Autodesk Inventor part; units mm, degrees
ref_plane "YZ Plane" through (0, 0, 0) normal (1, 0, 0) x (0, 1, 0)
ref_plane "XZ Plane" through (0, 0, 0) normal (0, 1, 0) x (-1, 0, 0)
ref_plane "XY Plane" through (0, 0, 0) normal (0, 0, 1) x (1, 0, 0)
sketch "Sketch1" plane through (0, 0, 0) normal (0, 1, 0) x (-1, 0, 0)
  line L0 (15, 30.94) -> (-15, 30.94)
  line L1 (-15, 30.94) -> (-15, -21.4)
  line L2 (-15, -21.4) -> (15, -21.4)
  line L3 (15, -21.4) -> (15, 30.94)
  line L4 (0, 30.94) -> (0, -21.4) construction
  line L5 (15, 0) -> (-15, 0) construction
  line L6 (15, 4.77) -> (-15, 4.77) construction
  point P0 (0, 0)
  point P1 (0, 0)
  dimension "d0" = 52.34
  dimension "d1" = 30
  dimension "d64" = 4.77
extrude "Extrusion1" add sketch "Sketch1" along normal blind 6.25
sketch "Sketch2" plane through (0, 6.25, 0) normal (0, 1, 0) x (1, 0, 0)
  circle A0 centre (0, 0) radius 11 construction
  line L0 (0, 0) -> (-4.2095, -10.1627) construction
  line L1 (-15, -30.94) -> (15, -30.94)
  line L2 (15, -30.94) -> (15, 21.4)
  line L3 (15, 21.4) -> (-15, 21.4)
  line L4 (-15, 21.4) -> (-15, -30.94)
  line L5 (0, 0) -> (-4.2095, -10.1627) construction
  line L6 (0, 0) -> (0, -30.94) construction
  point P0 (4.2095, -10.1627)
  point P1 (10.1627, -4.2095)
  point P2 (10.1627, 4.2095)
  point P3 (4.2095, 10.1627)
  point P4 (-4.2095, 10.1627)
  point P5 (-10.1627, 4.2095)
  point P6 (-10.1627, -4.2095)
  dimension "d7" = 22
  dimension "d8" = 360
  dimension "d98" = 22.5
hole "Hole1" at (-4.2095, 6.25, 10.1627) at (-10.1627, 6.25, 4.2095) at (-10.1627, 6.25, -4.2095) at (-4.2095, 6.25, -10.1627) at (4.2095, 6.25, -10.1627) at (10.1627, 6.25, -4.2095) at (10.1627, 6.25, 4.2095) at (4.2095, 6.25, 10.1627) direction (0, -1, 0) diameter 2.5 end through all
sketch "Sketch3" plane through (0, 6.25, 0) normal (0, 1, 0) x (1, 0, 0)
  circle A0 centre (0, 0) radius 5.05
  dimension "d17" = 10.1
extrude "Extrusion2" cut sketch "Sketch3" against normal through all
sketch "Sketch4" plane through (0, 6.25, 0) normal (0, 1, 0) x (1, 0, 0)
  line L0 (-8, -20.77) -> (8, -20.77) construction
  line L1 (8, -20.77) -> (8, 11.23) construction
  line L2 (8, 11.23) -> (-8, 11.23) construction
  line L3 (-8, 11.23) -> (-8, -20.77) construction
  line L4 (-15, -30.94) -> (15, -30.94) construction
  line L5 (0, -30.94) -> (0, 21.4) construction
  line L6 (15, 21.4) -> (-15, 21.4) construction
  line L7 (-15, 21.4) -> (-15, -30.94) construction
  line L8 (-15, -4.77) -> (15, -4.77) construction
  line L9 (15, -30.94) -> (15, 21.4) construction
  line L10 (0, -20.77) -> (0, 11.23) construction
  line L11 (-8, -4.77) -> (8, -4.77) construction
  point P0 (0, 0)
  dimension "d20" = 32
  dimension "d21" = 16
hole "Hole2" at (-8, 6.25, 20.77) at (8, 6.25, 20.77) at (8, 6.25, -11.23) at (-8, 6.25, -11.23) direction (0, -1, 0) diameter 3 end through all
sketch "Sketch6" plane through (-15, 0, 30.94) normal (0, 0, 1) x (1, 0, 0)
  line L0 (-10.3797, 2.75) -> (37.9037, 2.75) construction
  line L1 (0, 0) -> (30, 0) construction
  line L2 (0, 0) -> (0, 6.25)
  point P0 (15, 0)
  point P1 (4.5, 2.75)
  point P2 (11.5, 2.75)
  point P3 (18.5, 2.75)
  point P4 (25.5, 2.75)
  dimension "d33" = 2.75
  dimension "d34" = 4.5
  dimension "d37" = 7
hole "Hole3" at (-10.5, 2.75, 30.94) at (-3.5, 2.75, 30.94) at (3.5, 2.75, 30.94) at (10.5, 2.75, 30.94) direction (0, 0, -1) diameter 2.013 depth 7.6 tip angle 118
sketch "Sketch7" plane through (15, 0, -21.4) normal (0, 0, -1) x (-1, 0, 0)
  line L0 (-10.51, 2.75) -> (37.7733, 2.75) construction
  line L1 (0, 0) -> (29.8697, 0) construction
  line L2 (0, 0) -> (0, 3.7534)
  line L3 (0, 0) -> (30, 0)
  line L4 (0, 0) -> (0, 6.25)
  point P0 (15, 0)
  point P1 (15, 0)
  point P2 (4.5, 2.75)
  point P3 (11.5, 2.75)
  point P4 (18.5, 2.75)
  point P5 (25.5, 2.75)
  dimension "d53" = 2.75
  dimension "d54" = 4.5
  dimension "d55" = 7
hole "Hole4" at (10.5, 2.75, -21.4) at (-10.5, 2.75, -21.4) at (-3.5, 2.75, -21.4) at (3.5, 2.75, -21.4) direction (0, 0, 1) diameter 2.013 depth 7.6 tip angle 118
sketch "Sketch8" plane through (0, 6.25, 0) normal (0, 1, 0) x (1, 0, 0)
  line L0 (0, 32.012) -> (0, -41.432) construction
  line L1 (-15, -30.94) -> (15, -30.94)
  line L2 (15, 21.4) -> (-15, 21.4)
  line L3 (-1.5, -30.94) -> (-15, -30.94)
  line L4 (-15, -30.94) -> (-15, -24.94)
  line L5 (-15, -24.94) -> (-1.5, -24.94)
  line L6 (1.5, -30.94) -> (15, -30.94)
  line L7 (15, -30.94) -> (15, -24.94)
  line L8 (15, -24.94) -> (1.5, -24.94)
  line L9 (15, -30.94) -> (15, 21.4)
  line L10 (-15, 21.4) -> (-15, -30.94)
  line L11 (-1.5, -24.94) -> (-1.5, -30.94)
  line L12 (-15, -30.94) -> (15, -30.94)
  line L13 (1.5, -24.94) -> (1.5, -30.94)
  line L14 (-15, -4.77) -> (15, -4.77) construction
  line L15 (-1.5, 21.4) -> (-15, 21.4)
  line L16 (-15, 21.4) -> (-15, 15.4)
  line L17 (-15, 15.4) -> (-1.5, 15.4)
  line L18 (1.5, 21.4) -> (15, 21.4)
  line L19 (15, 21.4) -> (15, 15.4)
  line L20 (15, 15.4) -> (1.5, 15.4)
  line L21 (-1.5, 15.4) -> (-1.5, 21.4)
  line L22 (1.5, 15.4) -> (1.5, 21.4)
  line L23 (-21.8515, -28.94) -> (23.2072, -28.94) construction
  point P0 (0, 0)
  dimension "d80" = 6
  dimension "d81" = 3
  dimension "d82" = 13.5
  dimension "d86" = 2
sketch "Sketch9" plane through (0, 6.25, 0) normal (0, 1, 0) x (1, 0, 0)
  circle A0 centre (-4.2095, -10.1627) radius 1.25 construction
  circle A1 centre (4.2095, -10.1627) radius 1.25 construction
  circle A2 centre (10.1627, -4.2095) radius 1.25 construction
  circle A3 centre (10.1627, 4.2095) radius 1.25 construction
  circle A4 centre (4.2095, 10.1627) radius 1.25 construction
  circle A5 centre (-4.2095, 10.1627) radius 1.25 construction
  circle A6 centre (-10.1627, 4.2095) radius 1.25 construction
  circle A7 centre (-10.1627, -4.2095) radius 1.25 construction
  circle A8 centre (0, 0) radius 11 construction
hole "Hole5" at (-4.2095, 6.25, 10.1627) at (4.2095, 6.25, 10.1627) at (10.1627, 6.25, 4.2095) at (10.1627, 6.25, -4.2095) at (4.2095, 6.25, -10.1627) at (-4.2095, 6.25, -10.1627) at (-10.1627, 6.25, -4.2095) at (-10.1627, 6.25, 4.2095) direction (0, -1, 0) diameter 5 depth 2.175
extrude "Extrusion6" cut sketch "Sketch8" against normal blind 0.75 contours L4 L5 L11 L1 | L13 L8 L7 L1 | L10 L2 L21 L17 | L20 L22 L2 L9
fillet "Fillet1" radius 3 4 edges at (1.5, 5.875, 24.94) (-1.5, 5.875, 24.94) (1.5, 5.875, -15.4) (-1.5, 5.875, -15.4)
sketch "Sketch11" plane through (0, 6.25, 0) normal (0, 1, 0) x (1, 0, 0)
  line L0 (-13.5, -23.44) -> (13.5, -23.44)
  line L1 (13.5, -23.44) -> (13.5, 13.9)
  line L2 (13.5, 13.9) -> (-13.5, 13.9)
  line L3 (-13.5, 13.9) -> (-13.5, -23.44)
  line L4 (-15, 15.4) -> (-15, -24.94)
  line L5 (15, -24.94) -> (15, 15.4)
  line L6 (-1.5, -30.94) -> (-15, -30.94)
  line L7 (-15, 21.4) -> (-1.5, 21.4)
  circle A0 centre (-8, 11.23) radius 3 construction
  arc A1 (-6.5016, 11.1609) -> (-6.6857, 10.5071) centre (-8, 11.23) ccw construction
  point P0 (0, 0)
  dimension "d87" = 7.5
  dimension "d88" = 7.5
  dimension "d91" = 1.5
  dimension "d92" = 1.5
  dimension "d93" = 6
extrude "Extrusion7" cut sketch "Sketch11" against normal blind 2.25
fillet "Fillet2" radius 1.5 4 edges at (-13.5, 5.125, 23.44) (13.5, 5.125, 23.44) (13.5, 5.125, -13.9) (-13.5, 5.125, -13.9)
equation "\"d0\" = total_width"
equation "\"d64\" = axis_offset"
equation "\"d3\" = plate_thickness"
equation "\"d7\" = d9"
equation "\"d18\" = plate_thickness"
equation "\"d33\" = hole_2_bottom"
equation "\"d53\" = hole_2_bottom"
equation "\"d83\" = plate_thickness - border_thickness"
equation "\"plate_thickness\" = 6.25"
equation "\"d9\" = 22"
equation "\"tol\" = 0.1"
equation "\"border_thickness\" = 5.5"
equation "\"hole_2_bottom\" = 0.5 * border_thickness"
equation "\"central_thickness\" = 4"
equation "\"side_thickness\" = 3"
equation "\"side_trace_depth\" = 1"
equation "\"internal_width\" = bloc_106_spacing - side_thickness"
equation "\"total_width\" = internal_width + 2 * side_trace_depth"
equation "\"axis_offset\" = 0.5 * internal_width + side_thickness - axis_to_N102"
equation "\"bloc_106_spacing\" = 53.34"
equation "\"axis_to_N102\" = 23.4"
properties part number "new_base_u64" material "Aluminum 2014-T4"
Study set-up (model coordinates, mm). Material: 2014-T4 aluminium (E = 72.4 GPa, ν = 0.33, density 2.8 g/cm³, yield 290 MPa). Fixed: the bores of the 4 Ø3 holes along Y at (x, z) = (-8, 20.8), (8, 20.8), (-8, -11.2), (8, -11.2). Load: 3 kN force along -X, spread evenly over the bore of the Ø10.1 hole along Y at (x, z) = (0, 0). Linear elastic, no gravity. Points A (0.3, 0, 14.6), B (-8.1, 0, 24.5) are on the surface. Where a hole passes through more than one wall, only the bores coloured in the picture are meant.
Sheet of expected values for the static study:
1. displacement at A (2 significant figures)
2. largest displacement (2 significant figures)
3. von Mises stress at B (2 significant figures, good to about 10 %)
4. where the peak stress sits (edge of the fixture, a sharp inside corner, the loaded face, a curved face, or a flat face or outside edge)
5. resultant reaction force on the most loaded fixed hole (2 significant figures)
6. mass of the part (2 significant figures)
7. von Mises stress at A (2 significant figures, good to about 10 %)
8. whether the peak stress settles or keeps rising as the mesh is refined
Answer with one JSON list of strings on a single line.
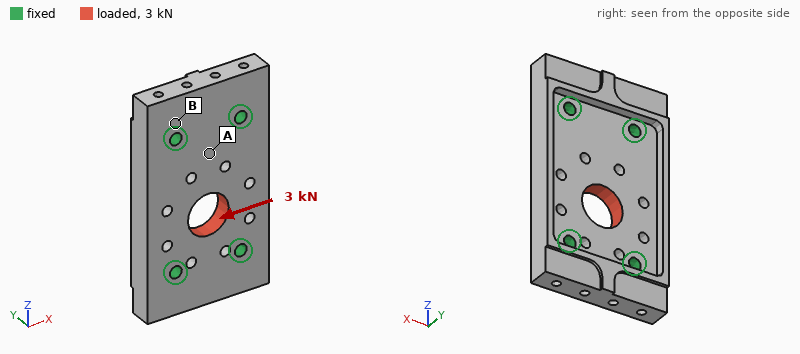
["2.9 µm", "10 µm", "7.3 MPa", "edge of the fixture", "950 N", "18 g", "18 MPa", "keeps rising"]
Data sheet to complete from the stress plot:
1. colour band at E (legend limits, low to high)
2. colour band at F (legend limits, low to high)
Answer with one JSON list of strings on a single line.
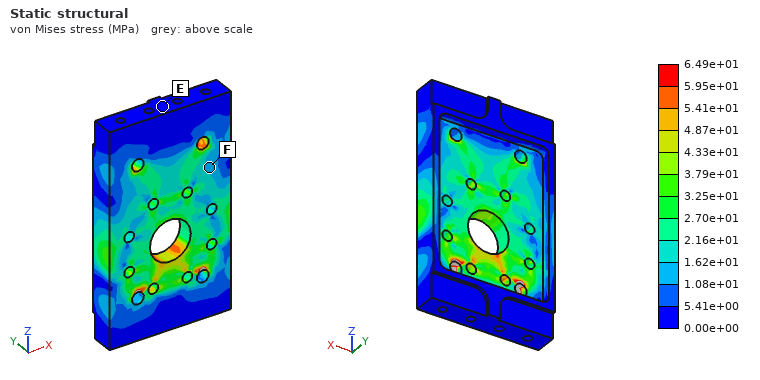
["0.00e+00 to 5.41e+00 MPa", "1.08e+01 to 1.62e+01 MPa"]
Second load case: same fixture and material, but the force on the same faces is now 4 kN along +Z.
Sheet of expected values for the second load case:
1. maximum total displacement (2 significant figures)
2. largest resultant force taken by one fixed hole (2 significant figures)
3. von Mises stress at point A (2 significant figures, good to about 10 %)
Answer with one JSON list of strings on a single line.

["6.2 µm", "1.2 kN", "20 MPa"]
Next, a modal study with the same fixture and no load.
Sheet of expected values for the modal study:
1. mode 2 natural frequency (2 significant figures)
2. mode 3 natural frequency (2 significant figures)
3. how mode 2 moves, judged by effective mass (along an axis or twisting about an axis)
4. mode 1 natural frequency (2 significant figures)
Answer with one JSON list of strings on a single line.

["21 kHz", "24 kHz", "twisting about Z", "18 kHz"]
